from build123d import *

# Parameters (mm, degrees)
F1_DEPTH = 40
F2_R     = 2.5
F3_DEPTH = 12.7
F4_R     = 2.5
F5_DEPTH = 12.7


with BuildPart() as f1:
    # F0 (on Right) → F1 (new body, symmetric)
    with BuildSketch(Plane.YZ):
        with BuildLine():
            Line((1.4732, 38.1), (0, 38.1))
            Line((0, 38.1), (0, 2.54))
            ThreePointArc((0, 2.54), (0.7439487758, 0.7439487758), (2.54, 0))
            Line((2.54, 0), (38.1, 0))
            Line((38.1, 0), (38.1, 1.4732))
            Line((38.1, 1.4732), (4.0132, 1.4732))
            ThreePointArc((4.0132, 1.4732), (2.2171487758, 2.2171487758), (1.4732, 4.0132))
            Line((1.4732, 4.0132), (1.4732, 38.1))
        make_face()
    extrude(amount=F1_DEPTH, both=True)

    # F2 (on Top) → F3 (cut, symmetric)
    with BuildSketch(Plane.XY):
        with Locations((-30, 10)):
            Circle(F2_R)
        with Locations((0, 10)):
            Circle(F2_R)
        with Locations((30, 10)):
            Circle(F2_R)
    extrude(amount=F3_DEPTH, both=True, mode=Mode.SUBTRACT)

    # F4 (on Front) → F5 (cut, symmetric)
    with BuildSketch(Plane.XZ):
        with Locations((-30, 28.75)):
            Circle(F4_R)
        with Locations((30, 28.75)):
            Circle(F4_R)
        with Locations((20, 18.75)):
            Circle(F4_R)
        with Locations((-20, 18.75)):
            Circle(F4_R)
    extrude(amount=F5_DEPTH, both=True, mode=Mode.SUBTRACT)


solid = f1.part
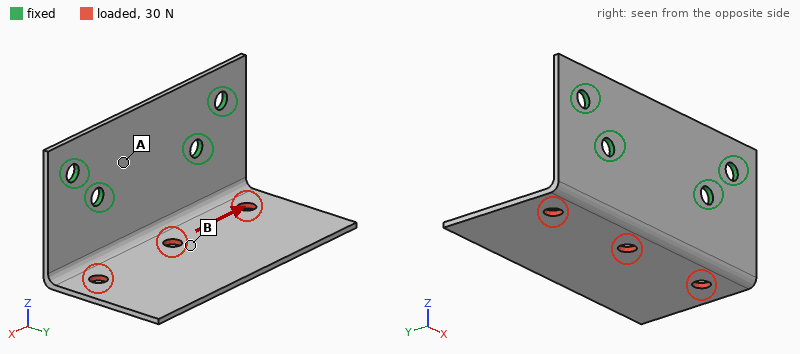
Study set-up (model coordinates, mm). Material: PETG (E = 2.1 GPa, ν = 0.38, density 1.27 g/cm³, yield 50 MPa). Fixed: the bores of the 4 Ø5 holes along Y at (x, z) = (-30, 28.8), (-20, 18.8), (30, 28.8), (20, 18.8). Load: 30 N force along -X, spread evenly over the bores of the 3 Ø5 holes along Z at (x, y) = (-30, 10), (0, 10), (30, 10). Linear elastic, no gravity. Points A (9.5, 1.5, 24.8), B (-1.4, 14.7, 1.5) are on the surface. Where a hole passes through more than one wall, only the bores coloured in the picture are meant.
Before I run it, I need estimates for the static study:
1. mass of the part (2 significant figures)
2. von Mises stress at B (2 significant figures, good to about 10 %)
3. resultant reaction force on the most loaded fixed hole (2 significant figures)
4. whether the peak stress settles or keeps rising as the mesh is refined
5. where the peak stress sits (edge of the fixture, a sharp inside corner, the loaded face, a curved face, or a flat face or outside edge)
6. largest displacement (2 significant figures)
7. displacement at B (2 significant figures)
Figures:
11 g
0.99 MPa
16 N
keeps rising
edge of the fixture
0.98 mm
0.21 mm
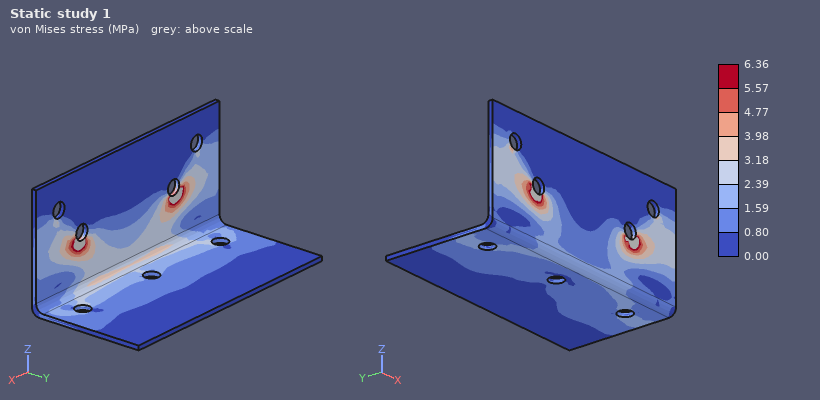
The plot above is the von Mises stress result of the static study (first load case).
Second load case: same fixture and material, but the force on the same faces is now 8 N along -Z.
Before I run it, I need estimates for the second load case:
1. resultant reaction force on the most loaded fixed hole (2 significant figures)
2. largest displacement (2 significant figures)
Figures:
2.9 N
1.1 mm
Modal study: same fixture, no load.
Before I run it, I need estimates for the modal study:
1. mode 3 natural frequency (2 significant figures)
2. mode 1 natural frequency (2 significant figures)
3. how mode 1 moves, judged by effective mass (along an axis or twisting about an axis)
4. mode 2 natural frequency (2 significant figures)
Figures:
390 Hz
130 Hz
along Z
220 Hz
